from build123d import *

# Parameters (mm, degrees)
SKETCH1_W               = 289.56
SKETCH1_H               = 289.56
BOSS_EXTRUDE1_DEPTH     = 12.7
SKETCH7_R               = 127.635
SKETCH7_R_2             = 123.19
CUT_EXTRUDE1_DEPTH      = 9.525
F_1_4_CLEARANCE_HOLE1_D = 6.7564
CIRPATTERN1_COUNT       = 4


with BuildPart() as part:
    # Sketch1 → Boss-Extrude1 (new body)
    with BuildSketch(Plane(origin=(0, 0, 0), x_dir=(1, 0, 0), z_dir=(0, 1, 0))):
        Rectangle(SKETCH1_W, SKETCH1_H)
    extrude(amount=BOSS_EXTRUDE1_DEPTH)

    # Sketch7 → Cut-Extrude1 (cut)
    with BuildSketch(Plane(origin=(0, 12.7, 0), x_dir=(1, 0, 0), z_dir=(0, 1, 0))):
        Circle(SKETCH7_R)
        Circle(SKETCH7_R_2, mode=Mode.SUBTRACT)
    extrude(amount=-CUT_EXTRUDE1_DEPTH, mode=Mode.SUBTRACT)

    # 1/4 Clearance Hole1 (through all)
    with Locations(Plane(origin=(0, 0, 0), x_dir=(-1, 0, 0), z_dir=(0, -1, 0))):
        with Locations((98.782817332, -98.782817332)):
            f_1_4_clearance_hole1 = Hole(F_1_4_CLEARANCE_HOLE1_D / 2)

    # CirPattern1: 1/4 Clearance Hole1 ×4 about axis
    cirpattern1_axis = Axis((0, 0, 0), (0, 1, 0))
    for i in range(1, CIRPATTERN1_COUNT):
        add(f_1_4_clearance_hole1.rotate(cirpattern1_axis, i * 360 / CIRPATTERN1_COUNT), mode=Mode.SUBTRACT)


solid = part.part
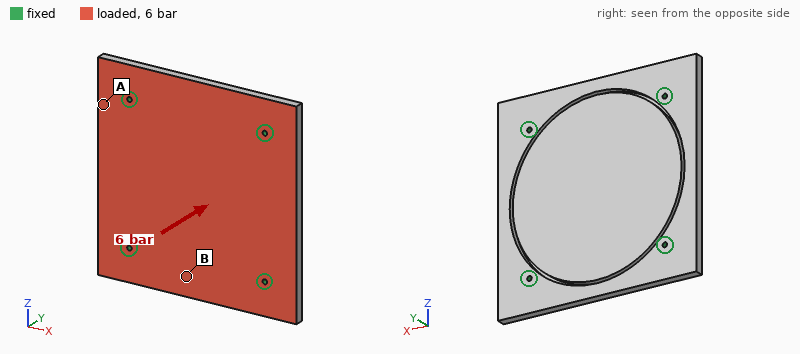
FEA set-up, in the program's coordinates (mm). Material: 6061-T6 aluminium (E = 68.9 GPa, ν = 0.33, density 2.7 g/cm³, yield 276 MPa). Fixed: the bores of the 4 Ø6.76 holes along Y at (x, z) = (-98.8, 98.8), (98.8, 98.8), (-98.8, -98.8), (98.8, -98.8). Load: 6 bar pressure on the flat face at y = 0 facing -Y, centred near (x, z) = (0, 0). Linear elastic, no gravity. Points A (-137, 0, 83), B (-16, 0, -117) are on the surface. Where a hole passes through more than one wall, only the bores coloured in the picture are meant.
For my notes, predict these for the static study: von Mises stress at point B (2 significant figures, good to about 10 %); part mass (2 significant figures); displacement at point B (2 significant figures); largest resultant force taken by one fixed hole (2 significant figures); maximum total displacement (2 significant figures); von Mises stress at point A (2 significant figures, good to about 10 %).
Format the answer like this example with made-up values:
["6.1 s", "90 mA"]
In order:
["61 MPa", "2.8 kg", "0.37 mm", "16 kN", "0.76 mm", "27 MPa"]
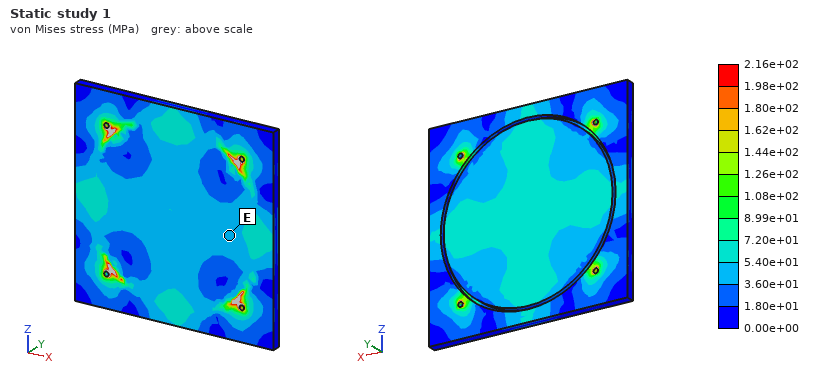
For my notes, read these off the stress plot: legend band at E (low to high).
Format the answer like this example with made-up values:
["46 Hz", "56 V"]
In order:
["3.60e+01 to 5.40e+01 MPa"]
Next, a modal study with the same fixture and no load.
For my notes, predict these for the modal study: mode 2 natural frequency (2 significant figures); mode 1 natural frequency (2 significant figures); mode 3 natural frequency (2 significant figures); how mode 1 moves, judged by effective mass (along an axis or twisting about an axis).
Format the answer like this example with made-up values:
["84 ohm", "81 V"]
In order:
["1300 Hz", "920 Hz", "1400 Hz", "along Y"]
